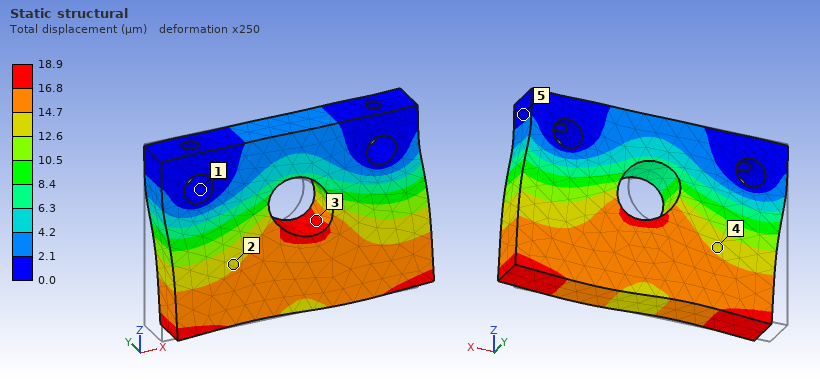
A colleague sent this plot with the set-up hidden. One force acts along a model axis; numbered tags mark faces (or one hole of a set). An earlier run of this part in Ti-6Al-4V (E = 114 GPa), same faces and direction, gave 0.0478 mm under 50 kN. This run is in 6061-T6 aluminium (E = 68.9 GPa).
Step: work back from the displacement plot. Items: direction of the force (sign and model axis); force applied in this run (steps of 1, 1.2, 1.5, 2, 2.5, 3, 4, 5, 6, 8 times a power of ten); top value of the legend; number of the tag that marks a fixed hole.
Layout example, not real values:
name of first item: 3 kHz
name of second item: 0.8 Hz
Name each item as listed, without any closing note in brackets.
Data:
direction of the force: +X
force applied in this run: 12 kN
top value of the legend: 18.9 µm
number of the tag that marks a fixed hole: 1
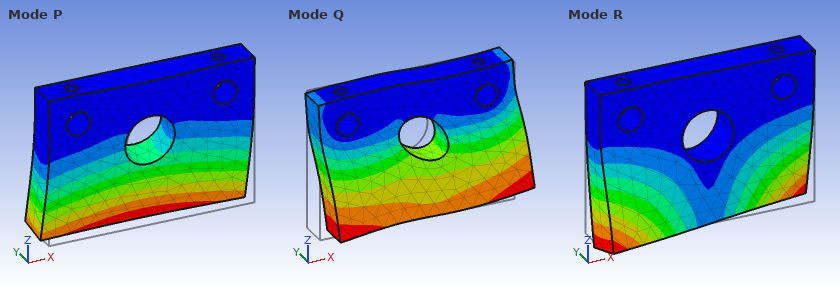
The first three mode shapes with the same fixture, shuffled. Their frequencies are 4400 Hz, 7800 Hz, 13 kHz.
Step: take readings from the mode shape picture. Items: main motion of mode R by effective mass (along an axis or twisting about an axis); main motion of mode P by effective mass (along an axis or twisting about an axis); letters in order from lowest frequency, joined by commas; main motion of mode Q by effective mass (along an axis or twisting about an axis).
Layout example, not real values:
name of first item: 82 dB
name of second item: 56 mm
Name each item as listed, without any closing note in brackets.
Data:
main motion of mode R by effective mass: twisting about Z
main motion of mode P by effective mass: along Y
letters in order from lowest frequency, joined by commas: P, R, Q
main motion of mode Q by effective mass: along X
